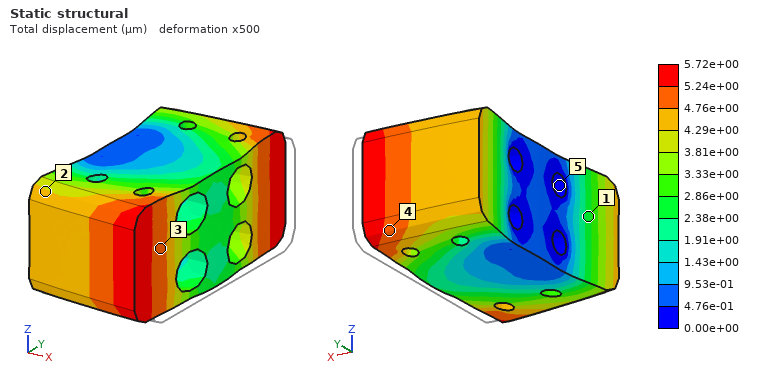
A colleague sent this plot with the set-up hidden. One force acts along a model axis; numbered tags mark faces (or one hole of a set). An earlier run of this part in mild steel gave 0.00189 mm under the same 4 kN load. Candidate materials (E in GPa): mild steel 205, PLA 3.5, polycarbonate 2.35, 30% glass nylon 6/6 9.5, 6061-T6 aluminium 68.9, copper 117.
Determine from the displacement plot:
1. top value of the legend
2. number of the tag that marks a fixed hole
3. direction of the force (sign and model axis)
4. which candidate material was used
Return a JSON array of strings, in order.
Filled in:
["5.72e+00 µm", "5", "-X", "6061-T6 aluminium"]
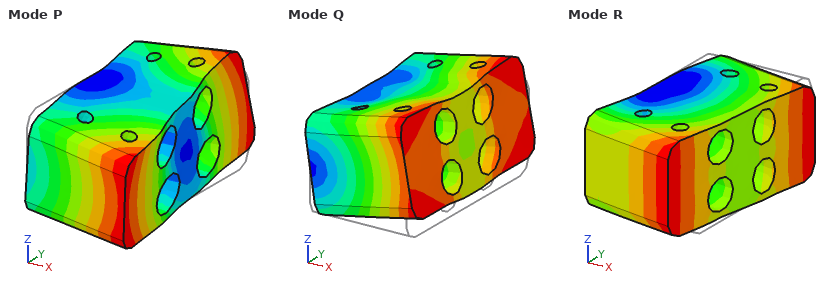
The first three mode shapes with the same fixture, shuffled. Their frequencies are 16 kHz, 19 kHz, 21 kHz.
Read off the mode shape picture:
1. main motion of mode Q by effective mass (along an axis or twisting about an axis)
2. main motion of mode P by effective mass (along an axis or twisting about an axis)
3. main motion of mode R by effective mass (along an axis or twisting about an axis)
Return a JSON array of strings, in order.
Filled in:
["along Z", "twisting about X", "along Y"]
